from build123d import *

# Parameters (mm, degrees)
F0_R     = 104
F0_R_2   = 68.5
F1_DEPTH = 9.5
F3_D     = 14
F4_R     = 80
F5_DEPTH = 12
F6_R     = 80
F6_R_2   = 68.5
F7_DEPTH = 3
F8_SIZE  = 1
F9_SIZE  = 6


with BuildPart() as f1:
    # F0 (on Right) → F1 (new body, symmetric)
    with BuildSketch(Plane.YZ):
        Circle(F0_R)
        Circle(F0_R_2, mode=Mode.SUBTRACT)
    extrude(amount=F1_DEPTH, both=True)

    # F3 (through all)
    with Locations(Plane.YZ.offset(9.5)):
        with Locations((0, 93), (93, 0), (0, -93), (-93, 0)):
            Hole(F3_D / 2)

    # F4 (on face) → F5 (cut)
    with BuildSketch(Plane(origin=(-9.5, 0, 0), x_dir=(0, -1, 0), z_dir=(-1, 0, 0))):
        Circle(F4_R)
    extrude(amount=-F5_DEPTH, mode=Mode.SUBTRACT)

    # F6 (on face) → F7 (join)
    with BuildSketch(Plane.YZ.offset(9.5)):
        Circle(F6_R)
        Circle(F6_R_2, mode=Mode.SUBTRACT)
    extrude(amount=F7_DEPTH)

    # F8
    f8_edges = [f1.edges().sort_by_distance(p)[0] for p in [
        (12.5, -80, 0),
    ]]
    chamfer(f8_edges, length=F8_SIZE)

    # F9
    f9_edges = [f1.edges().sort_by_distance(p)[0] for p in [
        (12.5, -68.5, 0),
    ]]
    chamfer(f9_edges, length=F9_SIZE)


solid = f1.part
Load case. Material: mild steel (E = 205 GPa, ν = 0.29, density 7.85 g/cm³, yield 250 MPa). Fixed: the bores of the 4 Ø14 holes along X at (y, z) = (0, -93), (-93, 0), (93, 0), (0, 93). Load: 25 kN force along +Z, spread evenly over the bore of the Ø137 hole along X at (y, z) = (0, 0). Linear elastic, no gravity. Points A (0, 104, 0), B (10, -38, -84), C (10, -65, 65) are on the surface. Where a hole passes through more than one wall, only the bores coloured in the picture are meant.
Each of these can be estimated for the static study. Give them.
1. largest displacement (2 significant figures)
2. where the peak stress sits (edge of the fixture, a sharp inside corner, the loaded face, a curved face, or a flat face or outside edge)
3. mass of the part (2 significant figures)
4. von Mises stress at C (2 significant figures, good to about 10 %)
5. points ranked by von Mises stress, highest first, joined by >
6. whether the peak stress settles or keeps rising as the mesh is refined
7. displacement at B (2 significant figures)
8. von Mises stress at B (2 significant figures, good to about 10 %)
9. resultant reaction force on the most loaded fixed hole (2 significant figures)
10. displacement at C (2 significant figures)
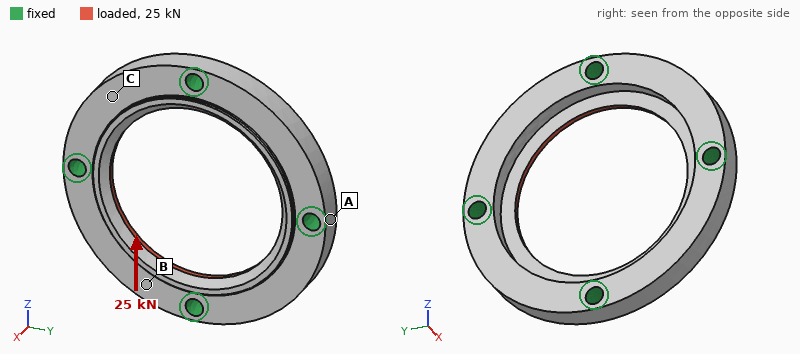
5.2 µm
edge of the fixture
2.3 kg
6.6 MPa
B > C > A
keeps rising
3.6 µm
8.4 MPa
8.1 kN
4.6 µm
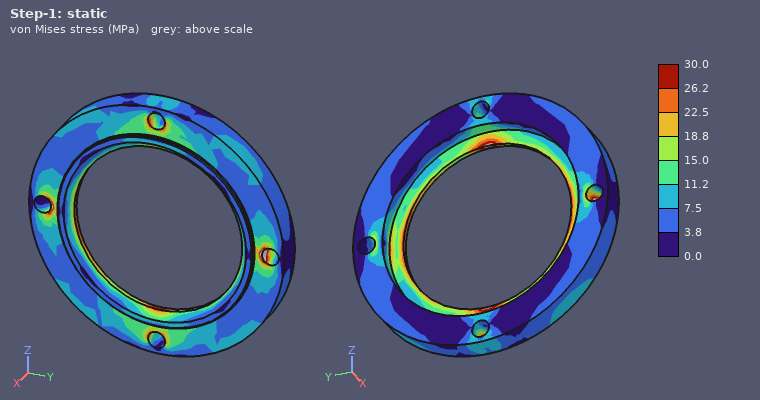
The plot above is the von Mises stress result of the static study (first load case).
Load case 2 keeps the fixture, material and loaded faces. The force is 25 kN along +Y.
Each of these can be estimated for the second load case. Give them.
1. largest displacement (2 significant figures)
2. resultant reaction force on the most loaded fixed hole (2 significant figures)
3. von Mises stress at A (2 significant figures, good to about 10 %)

5.2 µm
8.1 kN
7.1 MPa
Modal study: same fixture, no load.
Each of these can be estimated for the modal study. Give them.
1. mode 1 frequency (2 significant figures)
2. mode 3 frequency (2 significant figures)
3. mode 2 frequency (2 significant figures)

4500 Hz
4600 Hz
4600 Hz
